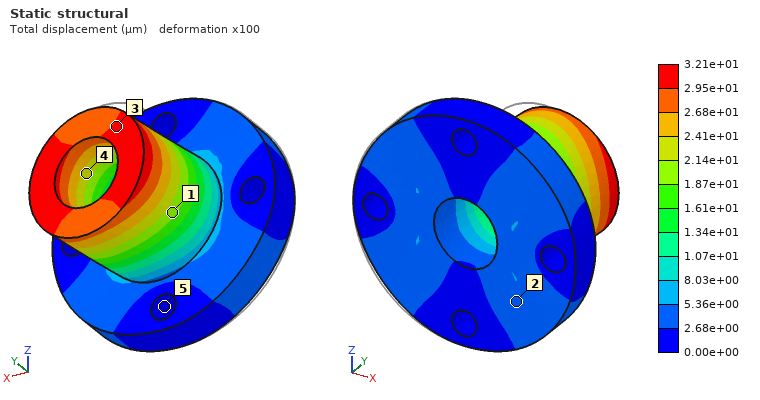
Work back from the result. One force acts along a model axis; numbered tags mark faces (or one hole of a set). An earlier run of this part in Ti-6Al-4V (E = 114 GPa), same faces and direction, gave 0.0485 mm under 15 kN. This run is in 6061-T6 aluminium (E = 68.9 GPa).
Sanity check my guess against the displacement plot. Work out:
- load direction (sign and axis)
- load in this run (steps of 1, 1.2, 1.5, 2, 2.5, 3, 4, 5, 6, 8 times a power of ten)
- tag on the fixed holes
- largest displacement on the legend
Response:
+X
6 kN
5
3.21e+01 µm
